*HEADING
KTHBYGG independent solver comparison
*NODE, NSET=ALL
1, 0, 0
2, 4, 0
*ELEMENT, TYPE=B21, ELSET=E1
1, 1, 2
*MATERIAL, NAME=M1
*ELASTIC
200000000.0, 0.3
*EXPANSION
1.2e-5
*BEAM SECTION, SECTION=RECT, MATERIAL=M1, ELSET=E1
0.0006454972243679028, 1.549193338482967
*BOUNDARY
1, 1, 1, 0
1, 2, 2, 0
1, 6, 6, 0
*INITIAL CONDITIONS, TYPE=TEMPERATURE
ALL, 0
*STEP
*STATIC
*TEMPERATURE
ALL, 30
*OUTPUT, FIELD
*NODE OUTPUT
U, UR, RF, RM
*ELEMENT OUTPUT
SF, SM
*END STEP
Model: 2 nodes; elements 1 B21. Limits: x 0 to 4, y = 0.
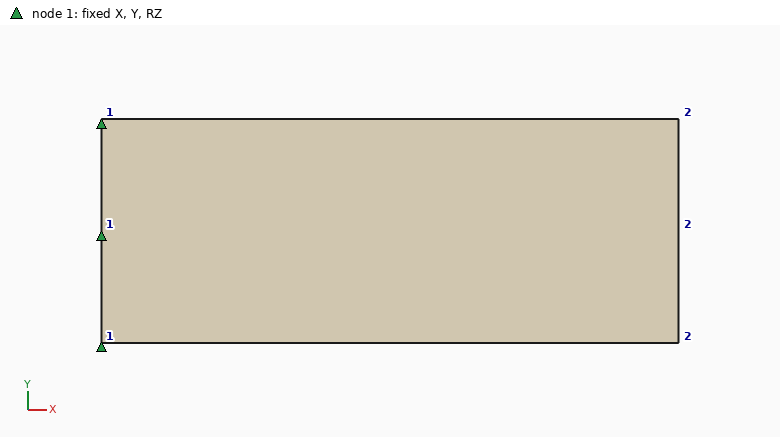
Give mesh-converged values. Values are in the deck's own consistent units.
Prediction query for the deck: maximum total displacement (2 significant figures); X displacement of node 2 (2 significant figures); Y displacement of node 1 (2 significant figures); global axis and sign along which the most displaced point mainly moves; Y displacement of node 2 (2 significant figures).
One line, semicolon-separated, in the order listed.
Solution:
0.0015; 0.0014; -2.8e-04; +X; 2.8e-04
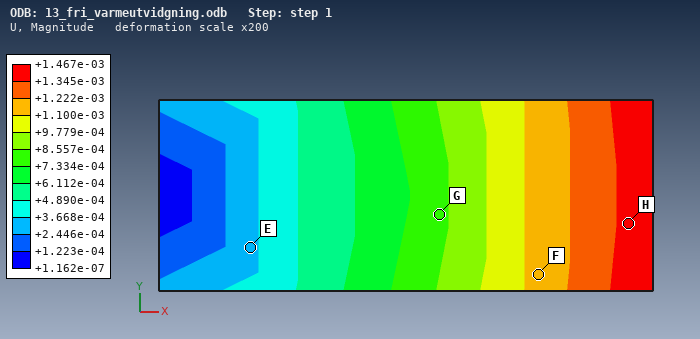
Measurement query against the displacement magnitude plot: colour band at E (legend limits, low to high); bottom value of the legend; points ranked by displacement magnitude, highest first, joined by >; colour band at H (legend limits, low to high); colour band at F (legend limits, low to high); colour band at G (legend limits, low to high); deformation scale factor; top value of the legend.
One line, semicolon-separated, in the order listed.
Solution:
+2.446e-04 to +3.668e-04; +1.162e-07; H > F > G > E; +1.345e-03 to +1.467e-03; +1.100e-03 to +1.222e-03; +7.334e-04 to +8.557e-04; 200; +1.467e-03
